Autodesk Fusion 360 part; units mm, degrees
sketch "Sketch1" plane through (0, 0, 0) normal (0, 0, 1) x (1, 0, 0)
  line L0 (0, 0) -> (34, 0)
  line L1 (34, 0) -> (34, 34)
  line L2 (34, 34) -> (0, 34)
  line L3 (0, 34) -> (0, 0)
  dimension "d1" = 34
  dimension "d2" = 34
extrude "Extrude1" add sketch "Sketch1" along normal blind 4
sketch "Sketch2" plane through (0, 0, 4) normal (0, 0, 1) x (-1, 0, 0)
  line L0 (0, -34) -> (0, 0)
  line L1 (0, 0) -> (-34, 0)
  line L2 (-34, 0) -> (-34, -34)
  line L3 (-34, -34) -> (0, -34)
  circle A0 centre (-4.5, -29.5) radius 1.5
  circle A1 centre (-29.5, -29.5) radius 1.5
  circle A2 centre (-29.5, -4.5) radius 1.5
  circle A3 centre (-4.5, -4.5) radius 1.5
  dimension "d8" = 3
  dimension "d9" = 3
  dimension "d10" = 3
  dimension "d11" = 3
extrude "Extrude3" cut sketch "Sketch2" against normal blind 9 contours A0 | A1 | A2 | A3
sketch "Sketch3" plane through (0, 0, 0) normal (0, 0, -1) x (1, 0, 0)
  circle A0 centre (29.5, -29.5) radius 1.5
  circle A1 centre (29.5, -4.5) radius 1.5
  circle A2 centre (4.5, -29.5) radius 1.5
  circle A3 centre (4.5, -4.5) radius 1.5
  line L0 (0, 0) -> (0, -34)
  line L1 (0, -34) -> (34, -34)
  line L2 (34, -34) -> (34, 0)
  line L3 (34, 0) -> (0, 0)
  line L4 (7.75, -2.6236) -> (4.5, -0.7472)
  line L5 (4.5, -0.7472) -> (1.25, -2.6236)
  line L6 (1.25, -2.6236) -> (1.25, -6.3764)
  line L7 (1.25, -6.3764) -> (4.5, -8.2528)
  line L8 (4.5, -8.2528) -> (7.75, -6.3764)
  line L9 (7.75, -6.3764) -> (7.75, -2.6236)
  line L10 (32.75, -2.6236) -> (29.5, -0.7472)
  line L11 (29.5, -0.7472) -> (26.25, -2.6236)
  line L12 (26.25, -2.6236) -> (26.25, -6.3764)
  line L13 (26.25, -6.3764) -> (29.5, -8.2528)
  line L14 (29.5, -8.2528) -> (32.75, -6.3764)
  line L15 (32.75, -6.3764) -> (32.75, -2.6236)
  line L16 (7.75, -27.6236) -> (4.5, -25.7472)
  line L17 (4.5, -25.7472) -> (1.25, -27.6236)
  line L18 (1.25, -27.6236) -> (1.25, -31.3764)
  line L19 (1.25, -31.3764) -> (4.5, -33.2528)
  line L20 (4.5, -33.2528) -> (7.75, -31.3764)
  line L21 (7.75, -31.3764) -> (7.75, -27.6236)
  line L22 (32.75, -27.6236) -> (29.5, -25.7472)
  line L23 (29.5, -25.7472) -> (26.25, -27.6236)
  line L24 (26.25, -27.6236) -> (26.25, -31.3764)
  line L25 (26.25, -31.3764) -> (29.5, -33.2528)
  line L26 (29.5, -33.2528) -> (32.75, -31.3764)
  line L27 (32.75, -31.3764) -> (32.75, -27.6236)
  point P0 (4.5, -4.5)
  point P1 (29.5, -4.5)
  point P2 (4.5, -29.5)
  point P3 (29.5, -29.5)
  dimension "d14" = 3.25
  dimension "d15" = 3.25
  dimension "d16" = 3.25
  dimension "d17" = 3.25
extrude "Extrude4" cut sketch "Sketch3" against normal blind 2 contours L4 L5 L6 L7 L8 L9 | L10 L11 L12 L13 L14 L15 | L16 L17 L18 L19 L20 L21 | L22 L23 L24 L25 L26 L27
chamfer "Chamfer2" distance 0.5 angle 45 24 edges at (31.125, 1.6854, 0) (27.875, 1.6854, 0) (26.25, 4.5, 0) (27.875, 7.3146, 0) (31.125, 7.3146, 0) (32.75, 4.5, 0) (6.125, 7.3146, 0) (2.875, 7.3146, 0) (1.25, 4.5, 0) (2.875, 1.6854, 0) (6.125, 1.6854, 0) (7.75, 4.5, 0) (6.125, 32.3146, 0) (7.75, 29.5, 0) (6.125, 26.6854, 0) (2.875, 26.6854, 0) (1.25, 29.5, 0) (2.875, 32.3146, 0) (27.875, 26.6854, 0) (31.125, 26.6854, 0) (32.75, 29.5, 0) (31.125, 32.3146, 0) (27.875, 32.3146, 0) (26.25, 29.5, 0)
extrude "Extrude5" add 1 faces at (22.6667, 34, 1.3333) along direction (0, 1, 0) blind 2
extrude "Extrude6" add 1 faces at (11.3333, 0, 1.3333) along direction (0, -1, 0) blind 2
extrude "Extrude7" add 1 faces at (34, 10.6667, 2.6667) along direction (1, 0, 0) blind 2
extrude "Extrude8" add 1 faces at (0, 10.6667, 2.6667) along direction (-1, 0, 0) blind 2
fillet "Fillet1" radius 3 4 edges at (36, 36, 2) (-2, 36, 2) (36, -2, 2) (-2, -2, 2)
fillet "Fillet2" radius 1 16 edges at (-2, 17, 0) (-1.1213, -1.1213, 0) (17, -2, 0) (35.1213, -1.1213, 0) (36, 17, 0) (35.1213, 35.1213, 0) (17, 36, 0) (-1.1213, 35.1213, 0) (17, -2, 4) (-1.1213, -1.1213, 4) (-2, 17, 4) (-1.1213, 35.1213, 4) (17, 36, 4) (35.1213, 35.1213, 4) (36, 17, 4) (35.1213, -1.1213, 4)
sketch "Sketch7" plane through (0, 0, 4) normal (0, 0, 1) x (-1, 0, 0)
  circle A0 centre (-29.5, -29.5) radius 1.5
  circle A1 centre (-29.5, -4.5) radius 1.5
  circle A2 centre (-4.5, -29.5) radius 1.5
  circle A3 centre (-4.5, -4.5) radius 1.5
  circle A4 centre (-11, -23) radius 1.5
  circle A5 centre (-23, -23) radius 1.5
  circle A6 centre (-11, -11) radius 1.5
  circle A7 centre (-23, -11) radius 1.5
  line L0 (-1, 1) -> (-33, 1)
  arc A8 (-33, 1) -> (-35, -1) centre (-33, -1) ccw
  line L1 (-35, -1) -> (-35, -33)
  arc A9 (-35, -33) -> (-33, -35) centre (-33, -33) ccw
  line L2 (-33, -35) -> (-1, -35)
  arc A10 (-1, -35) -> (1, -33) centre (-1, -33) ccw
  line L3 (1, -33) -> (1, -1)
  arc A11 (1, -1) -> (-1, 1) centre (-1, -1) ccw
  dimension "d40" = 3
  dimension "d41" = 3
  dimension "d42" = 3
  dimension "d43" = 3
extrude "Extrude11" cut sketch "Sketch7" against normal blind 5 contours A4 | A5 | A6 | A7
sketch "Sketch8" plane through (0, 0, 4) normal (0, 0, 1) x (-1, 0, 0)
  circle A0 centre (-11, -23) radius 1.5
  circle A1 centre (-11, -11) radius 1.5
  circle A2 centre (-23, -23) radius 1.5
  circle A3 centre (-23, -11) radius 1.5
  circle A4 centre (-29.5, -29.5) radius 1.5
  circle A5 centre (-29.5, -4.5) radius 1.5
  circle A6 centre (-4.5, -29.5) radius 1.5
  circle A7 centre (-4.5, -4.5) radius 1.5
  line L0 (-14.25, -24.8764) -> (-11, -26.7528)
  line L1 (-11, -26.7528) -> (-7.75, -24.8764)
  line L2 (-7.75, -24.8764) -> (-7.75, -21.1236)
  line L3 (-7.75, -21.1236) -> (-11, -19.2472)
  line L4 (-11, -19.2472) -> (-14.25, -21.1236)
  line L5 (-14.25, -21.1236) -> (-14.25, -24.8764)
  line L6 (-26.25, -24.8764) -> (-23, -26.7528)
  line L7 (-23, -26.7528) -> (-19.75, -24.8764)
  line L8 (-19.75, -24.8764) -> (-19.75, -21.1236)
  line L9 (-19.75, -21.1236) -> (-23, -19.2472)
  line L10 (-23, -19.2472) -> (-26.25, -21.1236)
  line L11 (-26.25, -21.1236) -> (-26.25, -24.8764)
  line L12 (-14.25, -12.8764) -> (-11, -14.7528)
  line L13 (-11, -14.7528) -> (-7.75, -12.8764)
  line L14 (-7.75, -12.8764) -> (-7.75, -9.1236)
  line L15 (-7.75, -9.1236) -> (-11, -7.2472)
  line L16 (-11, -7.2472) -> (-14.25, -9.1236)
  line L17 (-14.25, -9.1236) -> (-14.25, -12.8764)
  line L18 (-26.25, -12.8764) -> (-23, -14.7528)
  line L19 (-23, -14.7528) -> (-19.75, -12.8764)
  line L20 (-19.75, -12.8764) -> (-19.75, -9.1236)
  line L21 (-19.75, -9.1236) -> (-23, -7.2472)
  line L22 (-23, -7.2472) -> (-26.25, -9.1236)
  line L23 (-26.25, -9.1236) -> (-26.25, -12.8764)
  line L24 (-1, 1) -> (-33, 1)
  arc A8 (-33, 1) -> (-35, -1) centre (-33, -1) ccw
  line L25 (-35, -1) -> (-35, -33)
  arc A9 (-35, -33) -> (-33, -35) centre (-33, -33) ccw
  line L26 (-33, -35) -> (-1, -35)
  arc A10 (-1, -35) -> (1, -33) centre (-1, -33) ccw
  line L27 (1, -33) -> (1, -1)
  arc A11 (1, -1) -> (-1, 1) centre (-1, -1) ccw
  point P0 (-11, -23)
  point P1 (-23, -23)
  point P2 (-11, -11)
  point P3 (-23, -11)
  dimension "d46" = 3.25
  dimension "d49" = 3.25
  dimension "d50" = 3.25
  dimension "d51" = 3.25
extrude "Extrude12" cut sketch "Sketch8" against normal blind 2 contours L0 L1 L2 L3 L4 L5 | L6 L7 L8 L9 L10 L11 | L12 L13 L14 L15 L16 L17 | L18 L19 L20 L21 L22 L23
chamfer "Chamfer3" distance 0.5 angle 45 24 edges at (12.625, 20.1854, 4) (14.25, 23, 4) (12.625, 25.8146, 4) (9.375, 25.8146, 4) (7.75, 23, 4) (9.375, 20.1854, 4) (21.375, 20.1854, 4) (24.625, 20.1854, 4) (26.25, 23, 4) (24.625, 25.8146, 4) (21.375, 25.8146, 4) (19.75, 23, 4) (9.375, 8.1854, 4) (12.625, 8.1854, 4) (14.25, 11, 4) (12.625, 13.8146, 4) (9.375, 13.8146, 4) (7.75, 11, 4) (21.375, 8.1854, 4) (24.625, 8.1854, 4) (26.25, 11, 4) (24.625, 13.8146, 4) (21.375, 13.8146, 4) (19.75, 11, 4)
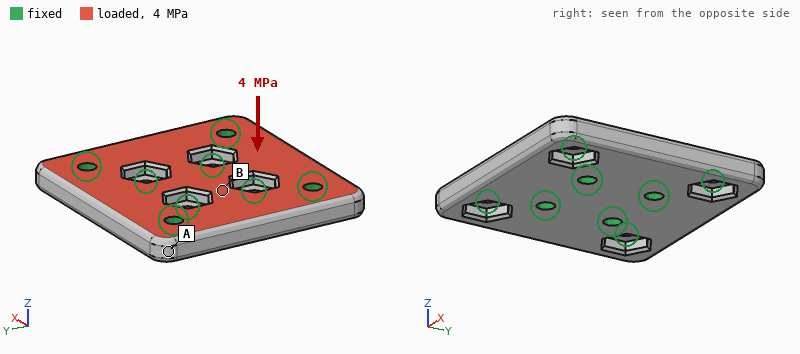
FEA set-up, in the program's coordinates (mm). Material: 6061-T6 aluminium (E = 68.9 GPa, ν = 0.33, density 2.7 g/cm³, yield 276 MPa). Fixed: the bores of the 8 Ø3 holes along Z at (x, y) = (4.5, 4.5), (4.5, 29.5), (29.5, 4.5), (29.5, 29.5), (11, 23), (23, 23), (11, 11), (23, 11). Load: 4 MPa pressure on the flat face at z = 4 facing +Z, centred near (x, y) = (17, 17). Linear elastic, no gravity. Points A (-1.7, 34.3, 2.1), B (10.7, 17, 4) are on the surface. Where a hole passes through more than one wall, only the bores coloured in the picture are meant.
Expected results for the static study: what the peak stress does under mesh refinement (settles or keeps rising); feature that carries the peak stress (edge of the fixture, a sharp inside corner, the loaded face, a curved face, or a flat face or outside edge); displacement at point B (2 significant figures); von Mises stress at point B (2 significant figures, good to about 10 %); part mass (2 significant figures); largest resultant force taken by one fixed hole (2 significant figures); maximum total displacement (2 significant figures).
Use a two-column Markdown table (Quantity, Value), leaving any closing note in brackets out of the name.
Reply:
| Quantity | Value |
|---|---|
| what the peak stress does under mesh refinement | keeps rising |
| feature that carries the peak stress | edge of the fixture |
| displacement at point B | 2.9 µm |
| von Mises stress at point B | 24 MPa |
| part mass | 13 g |
| largest resultant force taken by one fixed hole | 640 N |
| maximum total displacement | 16 µm |
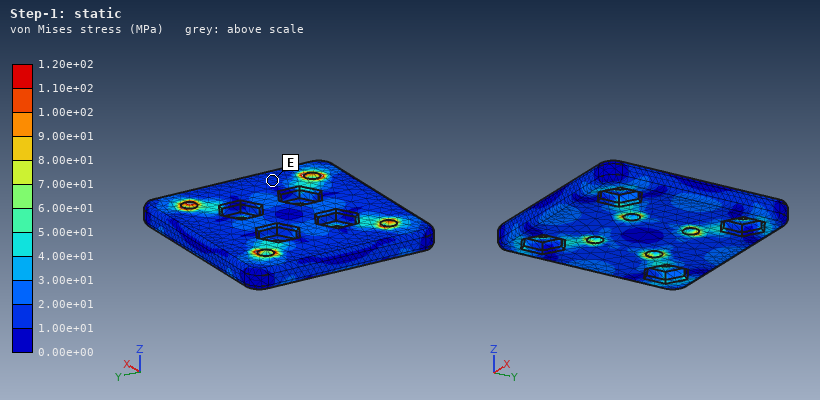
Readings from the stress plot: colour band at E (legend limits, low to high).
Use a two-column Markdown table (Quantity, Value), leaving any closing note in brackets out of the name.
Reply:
| Quantity | Value |
|---|---|
| colour band at E | 1.00e+01 to 2.00e+01 MPa |
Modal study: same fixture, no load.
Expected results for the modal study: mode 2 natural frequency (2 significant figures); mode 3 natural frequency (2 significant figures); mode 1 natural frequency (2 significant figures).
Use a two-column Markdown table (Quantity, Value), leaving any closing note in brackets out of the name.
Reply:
| Quantity | Value |
|---|---|
| mode 2 natural frequency | 26 kHz |
| mode 3 natural frequency | 26 kHz |
| mode 1 natural frequency | 24 kHz |
